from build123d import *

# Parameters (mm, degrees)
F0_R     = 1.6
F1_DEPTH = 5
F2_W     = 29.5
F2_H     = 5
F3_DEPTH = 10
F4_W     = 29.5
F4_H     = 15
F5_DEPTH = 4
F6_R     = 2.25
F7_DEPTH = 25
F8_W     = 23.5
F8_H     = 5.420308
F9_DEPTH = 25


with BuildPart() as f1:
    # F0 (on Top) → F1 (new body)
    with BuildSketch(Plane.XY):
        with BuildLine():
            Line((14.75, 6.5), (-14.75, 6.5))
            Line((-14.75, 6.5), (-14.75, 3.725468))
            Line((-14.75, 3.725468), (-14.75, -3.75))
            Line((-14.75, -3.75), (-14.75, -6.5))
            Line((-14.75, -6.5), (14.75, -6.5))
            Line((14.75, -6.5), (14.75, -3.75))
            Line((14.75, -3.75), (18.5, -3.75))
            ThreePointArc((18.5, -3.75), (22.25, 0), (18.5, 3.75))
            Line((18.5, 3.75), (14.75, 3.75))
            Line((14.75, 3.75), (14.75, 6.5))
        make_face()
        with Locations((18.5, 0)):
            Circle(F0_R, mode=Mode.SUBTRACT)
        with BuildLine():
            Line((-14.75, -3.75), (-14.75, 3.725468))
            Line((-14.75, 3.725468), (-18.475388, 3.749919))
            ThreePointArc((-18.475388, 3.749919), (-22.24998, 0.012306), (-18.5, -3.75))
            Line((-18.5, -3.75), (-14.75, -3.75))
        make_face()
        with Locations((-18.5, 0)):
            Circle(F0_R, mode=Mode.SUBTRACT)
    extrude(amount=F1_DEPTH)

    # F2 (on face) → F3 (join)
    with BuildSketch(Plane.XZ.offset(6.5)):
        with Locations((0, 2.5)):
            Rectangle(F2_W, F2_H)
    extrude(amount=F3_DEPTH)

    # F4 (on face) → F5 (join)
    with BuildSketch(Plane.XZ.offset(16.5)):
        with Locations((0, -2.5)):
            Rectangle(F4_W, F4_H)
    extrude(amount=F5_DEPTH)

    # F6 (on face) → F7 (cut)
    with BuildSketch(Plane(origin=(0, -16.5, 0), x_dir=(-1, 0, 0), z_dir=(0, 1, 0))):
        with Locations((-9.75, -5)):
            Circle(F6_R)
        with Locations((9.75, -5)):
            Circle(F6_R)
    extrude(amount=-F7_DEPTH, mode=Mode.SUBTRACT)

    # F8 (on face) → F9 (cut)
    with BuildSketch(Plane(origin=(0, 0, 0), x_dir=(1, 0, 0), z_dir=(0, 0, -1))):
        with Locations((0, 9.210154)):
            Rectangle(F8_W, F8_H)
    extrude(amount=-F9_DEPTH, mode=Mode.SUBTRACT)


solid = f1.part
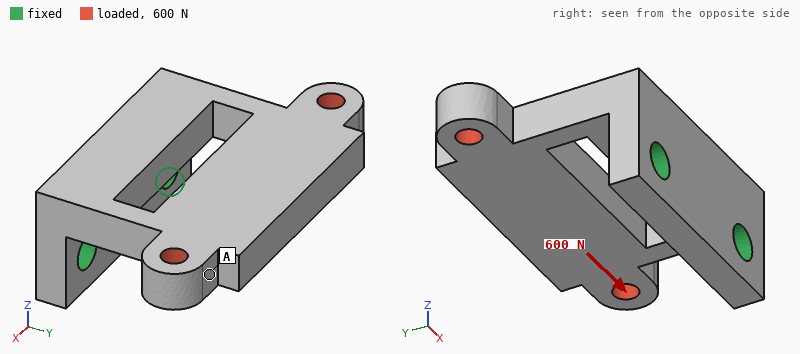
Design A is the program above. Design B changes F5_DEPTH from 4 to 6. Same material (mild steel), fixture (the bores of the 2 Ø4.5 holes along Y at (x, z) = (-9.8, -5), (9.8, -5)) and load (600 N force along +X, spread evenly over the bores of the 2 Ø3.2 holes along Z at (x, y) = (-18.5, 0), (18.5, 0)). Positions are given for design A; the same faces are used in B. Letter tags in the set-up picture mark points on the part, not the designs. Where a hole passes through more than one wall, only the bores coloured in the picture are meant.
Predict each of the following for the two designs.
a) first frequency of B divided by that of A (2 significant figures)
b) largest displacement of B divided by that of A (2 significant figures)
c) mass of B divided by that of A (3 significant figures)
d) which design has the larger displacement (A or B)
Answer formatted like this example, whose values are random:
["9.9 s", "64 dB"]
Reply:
["1.1", "0.80", "1.17", "A"]
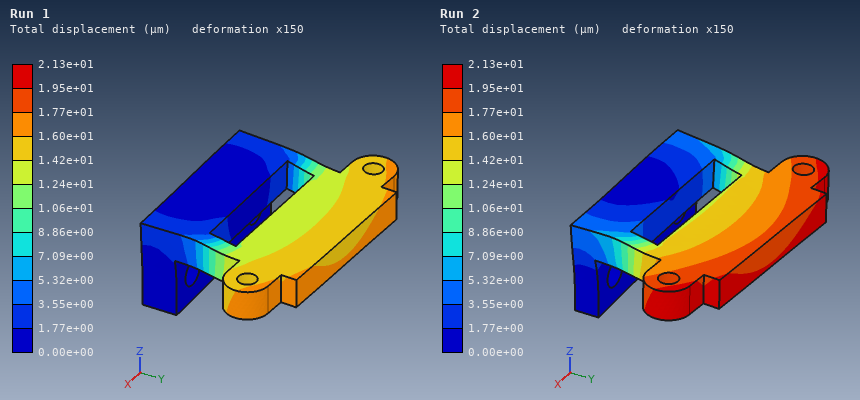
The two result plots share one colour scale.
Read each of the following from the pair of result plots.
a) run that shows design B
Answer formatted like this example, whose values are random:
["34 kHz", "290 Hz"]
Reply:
["Run 1"]
